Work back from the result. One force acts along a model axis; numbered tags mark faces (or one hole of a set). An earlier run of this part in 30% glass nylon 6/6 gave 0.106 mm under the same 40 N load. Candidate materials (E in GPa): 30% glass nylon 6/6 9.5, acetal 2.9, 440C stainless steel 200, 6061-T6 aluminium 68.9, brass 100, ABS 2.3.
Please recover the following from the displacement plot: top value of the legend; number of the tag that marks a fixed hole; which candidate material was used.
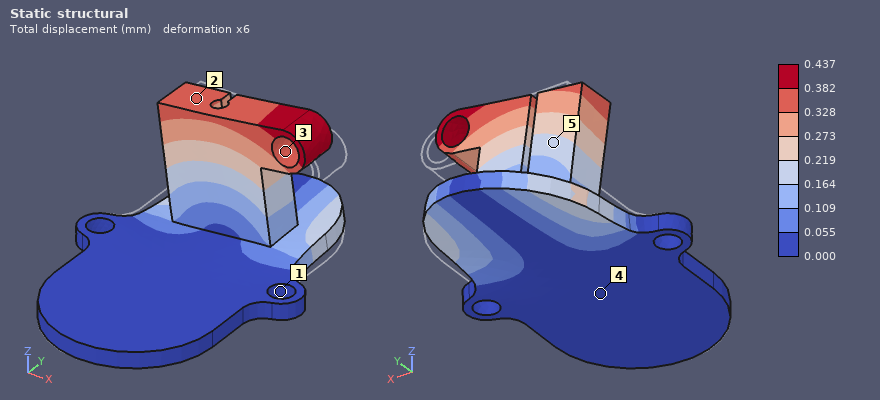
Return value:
0.437 mm
1
ABS
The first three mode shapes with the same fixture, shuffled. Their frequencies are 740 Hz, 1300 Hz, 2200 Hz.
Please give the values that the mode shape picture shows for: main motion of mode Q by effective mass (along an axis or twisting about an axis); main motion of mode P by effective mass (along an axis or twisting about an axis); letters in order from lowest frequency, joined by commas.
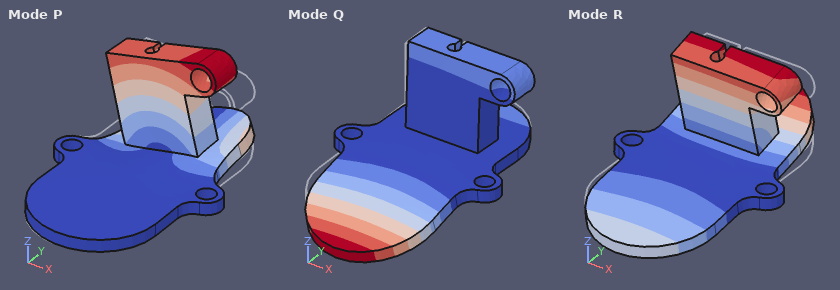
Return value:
along Z
along X
R, Q, P
